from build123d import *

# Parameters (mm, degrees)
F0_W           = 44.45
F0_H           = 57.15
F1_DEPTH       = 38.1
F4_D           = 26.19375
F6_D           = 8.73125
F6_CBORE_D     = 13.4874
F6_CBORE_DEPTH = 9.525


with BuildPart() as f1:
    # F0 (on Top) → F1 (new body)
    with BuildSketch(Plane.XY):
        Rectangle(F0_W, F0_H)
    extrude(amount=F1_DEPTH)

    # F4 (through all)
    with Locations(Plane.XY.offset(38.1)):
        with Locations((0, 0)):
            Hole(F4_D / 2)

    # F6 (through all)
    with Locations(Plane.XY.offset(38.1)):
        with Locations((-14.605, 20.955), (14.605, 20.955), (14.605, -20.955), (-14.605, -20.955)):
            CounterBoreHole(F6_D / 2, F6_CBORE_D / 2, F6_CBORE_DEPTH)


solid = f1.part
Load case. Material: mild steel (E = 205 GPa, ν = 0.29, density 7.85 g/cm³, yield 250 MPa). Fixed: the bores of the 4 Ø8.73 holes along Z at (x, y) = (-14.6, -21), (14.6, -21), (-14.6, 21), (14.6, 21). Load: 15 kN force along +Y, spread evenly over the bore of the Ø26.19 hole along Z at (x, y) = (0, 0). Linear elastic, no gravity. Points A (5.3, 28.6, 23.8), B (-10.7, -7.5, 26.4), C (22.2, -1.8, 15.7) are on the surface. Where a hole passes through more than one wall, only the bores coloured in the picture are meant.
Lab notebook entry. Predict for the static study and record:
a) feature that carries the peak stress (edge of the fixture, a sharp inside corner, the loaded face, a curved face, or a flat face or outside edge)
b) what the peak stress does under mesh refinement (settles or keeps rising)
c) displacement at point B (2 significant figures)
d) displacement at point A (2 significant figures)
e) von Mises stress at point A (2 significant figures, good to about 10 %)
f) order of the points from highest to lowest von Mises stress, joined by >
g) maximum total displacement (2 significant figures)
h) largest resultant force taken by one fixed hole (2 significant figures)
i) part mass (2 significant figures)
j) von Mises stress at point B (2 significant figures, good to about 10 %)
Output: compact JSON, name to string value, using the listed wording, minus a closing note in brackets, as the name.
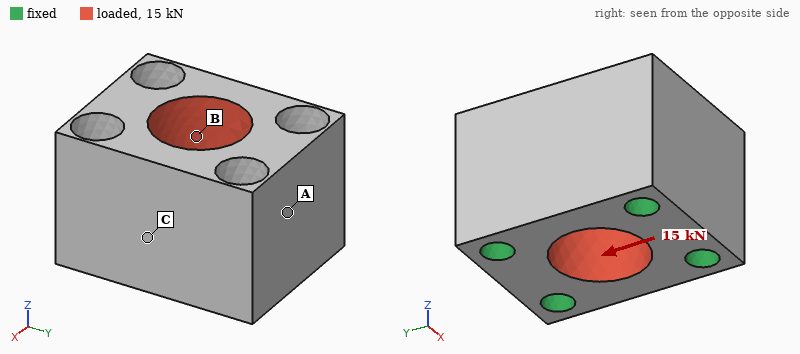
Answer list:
{"feature that carries the peak stress": "edge of the fixture", "what the peak stress does under mesh refinement": "keeps rising", "displacement at point B": "0.57 µm", "displacement at point A": "0.41 µm", "von Mises stress at point A": "5.5 MPa", "order of the points from highest to lowest von Mises stress, joined by >": "B > A > C", "maximum total displacement": "1.3 µm", "largest resultant force taken by one fixed hole": "3.8 kN", "part mass": "500 g", "von Mises stress at point B": "11 MPa"}
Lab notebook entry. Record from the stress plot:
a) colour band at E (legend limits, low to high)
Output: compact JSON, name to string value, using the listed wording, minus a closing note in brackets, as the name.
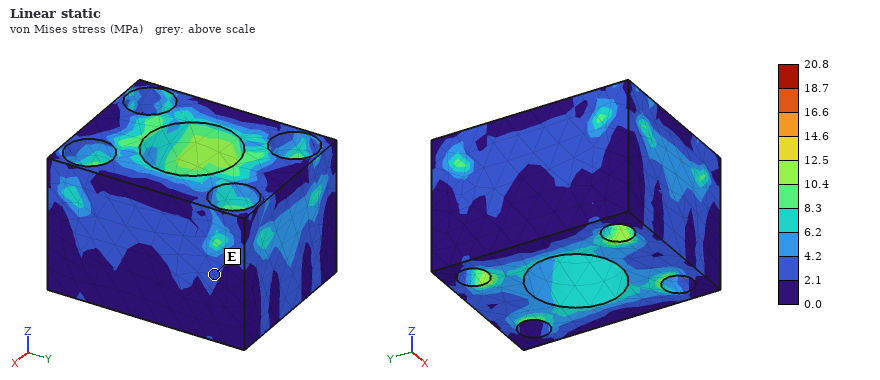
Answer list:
{"colour band at E": "2.1 to 4.2 MPa"}
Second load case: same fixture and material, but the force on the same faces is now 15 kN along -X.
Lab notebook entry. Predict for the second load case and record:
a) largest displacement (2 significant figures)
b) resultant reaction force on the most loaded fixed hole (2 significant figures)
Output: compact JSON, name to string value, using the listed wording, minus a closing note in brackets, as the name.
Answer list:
{"largest displacement": "2.1 µm", "resultant reaction force on the most loaded fixed hole": "3.9 kN"}
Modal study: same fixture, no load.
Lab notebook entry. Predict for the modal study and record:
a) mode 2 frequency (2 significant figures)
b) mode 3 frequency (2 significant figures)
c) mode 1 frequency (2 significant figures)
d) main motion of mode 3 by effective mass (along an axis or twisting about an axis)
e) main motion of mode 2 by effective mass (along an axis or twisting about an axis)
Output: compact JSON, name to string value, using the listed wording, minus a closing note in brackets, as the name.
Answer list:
{"mode 2 frequency": "32 kHz", "mode 3 frequency": "37 kHz", "mode 1 frequency": "30 kHz", "main motion of mode 3 by effective mass": "along Y", "main motion of mode 2 by effective mass": "along X"}
